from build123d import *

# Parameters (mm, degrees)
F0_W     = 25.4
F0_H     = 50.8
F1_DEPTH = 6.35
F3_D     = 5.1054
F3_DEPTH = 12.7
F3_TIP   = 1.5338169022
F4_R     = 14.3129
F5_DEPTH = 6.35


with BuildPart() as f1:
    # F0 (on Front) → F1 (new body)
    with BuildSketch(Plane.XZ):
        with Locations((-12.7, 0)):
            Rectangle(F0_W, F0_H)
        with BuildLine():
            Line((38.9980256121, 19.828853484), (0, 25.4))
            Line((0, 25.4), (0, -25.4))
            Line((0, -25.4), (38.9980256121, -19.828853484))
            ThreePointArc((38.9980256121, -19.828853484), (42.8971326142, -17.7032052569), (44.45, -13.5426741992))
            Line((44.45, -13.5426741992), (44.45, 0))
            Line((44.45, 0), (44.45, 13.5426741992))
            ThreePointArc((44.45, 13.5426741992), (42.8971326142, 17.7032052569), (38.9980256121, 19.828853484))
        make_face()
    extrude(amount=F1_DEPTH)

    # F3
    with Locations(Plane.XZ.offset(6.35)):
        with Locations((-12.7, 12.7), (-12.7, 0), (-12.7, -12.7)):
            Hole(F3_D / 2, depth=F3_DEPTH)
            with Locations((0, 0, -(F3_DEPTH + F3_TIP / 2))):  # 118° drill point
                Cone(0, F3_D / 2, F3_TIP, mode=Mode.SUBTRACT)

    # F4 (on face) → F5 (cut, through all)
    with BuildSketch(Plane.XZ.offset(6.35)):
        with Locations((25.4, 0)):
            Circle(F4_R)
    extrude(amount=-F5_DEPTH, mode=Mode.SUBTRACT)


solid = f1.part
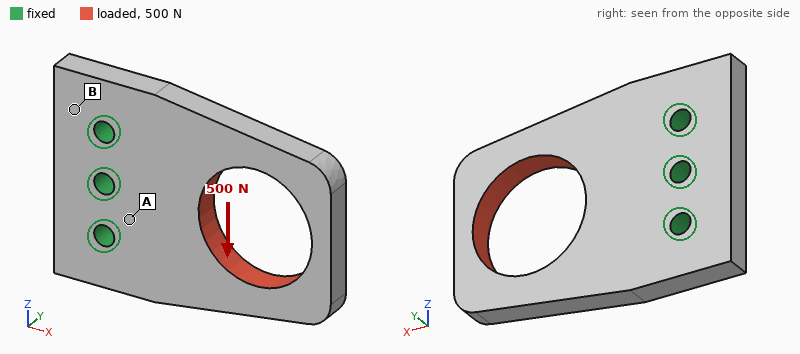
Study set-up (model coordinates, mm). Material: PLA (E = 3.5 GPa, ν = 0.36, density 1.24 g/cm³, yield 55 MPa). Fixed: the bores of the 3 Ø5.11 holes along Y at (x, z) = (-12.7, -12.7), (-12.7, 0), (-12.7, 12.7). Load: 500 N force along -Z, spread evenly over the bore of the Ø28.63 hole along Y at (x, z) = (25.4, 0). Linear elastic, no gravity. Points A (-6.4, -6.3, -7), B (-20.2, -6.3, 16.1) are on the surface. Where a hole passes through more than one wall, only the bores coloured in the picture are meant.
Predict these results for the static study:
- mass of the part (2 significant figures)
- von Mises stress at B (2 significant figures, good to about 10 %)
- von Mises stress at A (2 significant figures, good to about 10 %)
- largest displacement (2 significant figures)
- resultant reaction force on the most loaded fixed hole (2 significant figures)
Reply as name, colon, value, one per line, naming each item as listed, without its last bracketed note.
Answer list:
mass of the part: 20 g
von Mises stress at B: 2.8 MPa
von Mises stress at A: 6.2 MPa
largest displacement: 0.40 mm
resultant reaction force on the most loaded fixed hole: 660 N
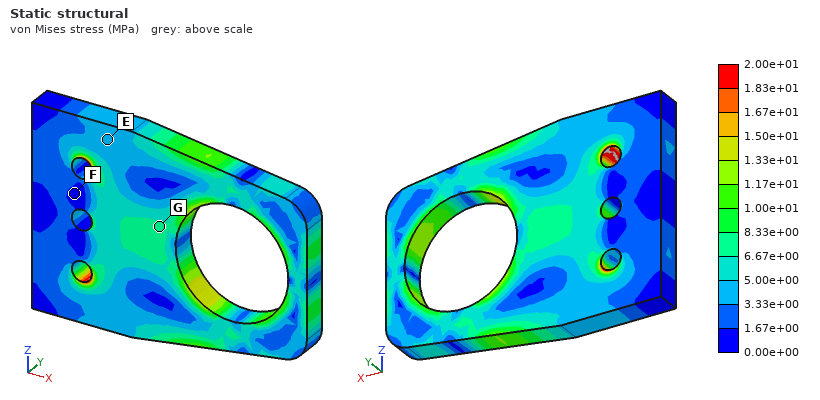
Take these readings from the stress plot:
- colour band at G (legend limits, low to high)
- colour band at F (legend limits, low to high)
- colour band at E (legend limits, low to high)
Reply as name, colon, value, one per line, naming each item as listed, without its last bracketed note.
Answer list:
colour band at G: 6.67e+00 to 8.33e+00 MPa
colour band at F: 0.00e+00 to 1.67e+00 MPa
colour band at E: 3.33e+00 to 5.00e+00 MPa
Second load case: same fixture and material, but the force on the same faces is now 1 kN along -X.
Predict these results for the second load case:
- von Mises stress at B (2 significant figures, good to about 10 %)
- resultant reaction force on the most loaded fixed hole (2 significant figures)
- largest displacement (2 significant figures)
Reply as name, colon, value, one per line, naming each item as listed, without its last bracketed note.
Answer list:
von Mises stress at B: 1.7 MPa
resultant reaction force on the most loaded fixed hole: 430 N
largest displacement: 0.19 mm
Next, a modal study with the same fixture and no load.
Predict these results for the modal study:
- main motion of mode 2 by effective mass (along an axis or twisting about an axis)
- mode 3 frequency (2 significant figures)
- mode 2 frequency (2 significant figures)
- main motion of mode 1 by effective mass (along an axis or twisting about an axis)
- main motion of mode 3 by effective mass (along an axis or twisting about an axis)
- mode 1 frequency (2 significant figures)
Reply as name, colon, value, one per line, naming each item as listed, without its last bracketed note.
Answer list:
main motion of mode 2 by effective mass: twisting about X
mode 3 frequency: 2400 Hz
mode 2 frequency: 1500 Hz
main motion of mode 1 by effective mass: along Y
main motion of mode 3 by effective mass: along Z
mode 1 frequency: 690 Hz
